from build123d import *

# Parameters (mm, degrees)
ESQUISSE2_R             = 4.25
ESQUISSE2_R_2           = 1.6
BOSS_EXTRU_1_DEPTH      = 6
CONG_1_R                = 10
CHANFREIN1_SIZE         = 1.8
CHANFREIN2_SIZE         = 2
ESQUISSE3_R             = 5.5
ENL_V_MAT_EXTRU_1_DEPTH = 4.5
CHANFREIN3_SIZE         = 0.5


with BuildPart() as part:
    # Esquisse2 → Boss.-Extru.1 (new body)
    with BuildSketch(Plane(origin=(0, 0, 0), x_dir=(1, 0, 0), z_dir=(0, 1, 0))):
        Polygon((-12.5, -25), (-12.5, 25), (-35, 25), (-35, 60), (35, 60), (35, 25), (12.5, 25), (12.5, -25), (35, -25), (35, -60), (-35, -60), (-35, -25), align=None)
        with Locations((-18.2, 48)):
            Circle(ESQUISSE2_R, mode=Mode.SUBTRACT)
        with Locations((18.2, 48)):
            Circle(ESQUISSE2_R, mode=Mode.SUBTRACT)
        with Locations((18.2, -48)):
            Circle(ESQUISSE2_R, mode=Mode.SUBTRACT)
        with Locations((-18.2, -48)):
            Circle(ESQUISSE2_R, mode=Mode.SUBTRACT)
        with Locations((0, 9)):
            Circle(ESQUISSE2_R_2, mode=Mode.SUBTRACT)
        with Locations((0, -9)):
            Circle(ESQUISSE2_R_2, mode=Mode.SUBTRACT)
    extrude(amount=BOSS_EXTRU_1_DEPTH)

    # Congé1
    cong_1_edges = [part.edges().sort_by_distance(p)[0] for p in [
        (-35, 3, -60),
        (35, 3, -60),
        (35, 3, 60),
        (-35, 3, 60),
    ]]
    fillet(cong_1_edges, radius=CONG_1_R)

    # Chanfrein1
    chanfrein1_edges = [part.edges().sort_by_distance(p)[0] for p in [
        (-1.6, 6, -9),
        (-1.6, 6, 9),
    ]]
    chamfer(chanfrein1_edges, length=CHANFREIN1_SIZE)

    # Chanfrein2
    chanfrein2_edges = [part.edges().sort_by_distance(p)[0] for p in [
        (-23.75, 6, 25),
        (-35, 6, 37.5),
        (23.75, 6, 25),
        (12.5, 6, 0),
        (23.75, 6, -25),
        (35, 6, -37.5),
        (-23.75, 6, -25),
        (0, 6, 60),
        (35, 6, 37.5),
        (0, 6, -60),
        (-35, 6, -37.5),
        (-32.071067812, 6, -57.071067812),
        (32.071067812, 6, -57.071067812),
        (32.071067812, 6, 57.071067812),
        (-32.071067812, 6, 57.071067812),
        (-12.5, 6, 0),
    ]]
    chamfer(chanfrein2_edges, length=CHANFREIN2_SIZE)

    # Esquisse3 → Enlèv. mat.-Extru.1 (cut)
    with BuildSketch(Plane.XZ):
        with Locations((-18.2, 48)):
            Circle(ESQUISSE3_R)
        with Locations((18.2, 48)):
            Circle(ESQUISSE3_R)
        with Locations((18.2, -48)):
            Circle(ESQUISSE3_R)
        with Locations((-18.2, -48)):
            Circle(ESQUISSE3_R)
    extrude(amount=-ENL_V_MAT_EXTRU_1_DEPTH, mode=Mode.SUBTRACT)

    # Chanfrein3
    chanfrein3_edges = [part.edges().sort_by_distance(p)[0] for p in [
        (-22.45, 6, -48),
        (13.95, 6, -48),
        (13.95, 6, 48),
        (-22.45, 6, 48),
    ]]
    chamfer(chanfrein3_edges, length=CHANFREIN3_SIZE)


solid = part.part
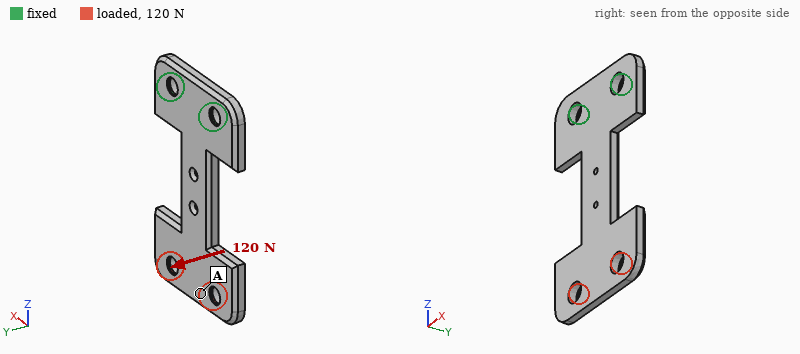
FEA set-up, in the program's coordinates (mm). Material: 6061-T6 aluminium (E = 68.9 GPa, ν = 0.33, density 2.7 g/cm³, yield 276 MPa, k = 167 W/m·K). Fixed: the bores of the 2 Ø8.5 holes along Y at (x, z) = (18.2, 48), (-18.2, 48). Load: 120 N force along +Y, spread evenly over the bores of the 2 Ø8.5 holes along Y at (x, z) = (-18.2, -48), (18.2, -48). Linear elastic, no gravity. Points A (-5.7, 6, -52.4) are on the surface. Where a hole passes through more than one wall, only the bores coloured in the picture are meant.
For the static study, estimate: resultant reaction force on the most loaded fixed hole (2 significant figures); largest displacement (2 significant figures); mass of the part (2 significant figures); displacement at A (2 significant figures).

190 N
1.4 mm
90 g
1.2 mm
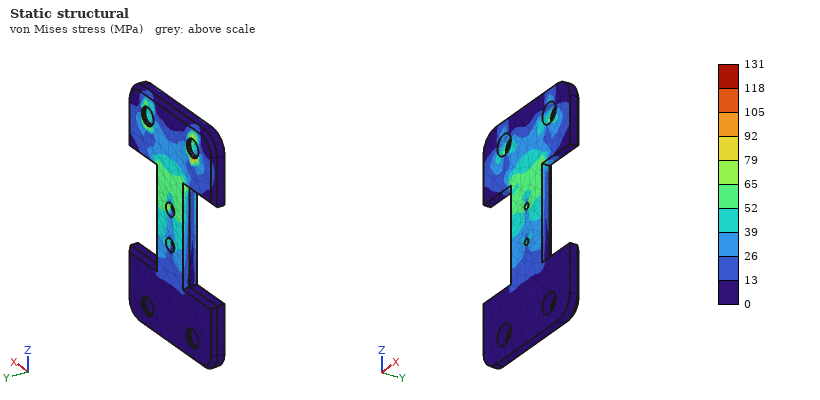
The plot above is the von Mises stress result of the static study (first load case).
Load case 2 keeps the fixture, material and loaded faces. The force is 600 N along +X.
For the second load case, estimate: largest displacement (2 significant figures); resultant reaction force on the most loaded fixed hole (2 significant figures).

0.33 mm
1.5 kN
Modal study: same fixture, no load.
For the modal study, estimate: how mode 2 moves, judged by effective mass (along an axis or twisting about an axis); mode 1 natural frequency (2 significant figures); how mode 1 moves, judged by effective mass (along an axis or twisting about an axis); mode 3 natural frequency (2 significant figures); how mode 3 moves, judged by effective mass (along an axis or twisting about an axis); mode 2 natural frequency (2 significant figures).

twisting about Z
280 Hz
along Y
1300 Hz
along X
990 Hz
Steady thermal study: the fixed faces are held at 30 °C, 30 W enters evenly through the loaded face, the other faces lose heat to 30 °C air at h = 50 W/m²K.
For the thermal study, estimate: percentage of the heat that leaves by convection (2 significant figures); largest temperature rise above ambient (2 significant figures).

60 %
56 K
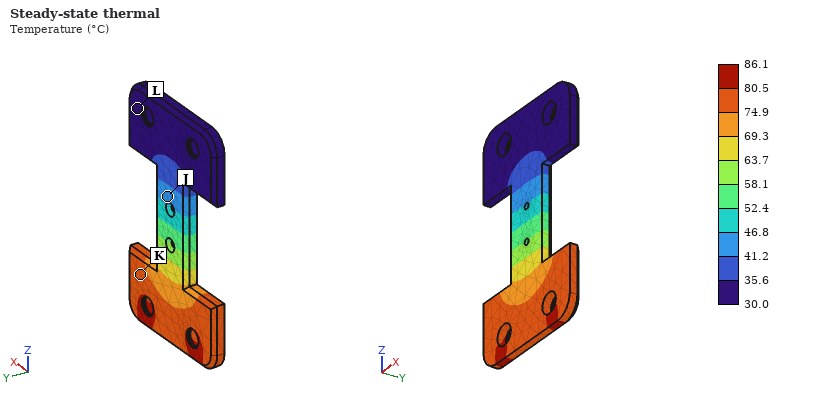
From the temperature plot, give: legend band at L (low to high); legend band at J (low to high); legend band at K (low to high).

30.0 to 35.6 °C
41.2 to 46.8 °C
74.9 to 80.5 °C
